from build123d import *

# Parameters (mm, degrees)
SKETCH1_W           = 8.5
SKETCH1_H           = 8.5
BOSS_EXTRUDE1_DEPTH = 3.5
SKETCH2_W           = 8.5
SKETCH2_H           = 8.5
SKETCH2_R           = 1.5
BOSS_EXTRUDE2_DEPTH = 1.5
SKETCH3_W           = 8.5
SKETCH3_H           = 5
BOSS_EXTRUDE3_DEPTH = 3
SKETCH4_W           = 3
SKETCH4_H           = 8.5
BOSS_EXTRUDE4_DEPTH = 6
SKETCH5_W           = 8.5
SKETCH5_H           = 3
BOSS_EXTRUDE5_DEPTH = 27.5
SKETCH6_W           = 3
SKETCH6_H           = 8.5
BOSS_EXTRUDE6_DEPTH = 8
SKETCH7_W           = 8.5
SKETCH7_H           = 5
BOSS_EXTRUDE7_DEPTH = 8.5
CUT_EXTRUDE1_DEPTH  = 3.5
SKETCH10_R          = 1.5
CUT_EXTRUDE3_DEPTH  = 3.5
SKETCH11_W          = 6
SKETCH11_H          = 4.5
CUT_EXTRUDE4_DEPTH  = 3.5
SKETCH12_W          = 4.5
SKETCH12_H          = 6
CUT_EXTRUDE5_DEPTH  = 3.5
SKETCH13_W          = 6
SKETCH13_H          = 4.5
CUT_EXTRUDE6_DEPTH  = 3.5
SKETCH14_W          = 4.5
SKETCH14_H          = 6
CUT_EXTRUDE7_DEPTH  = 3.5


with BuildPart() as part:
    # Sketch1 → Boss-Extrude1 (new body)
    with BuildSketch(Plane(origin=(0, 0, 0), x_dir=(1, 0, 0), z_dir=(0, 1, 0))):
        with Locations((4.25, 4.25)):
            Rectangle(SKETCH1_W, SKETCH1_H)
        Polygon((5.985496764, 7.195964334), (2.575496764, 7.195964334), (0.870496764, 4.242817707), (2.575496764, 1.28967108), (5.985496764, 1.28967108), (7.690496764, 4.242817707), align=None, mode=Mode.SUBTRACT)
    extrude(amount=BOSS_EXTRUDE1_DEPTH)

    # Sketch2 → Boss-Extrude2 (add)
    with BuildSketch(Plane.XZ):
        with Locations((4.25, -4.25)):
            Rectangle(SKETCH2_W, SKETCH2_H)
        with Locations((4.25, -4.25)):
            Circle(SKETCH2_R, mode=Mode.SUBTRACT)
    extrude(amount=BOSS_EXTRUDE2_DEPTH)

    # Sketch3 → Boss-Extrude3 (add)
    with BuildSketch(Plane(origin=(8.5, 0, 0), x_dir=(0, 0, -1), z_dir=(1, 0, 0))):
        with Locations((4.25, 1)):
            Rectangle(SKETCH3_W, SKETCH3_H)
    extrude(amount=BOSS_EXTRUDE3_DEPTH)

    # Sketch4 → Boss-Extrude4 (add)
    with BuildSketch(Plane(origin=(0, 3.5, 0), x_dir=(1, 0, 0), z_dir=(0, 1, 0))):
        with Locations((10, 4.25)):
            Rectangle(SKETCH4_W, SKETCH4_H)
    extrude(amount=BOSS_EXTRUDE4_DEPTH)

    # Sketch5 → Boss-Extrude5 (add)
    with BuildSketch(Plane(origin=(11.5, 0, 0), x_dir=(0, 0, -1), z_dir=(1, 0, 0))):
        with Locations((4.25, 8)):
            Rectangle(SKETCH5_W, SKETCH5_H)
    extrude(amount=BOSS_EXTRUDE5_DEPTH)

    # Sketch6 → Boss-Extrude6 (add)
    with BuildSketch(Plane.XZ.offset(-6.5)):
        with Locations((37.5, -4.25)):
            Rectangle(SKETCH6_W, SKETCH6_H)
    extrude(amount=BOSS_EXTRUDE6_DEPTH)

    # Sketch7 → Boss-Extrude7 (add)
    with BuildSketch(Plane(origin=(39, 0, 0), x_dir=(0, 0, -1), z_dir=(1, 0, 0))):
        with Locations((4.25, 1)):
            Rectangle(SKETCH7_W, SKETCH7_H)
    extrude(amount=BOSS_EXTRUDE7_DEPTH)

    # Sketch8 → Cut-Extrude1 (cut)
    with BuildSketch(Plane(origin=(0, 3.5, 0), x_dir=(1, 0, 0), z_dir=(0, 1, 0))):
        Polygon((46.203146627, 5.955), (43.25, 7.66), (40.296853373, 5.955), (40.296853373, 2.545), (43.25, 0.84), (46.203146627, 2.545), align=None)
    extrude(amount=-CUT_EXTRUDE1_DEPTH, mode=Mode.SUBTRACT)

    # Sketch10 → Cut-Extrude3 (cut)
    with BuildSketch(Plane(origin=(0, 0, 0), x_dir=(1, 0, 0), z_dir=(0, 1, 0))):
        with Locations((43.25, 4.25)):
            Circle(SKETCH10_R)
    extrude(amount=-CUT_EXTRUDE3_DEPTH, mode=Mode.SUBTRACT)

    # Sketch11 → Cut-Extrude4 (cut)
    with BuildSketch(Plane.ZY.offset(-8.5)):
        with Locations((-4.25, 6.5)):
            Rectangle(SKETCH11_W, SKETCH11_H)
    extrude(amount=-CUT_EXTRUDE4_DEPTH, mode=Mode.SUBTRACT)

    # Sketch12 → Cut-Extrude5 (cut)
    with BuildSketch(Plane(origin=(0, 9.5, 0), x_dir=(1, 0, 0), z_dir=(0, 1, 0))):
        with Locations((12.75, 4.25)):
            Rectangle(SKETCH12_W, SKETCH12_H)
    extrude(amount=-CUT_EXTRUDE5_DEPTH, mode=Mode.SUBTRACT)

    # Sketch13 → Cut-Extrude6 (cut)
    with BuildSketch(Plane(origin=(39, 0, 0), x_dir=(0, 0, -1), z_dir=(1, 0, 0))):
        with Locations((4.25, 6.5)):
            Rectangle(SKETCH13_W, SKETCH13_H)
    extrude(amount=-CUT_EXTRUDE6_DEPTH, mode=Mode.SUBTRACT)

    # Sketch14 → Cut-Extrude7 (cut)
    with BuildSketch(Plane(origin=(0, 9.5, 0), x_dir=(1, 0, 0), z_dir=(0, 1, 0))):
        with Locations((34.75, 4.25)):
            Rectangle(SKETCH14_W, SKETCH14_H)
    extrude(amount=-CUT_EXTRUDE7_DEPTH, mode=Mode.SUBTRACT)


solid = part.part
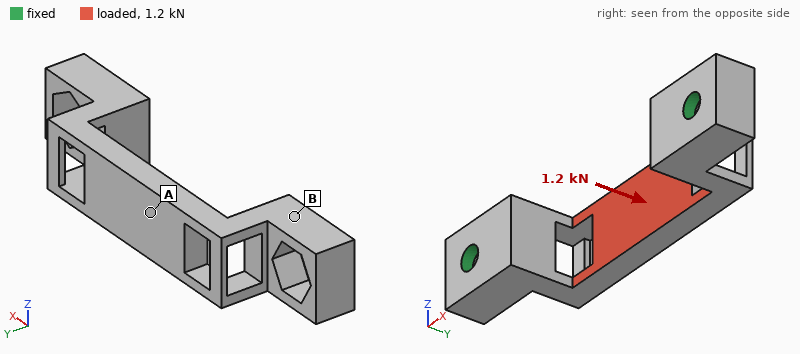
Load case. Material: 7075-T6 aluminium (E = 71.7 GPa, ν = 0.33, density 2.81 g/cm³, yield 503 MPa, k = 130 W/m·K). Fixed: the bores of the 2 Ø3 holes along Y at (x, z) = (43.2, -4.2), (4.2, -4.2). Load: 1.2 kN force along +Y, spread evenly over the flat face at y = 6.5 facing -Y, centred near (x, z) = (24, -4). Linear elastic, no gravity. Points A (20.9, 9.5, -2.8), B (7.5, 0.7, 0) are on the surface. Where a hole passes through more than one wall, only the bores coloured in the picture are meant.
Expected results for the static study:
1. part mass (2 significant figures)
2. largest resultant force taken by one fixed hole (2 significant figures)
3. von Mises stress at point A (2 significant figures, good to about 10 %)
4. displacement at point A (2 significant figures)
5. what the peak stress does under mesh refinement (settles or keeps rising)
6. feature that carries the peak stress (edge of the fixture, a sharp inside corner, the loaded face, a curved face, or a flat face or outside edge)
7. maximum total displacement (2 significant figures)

3.9 g
820 N
220 MPa
0.16 mm
keeps rising
a sharp inside corner
0.17 mm
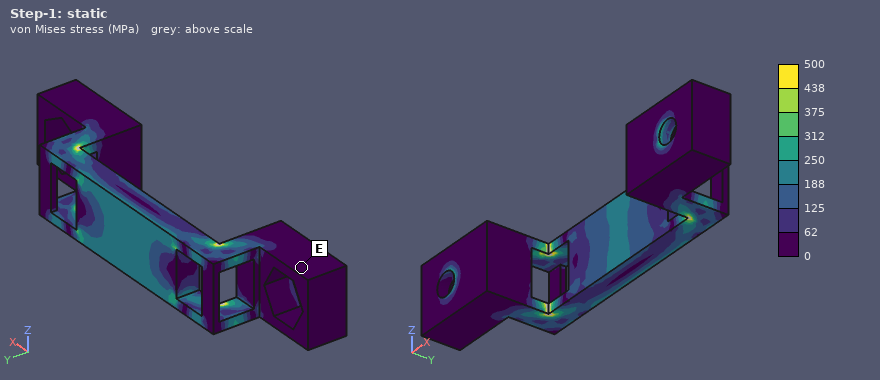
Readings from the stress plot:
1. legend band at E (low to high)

0 to 62 MPa
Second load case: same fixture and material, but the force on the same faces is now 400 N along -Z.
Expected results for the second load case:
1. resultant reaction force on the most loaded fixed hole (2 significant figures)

200 N
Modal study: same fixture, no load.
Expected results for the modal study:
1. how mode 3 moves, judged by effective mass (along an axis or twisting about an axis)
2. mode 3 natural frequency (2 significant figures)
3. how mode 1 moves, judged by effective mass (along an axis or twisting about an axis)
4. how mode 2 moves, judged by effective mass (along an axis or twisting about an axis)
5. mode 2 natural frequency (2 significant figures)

along Y
12 kHz
along Z
along X
11 kHz
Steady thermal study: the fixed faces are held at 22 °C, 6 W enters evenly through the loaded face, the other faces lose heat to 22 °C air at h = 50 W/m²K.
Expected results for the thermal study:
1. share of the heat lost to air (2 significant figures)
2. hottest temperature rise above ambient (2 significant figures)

15 %
33 K
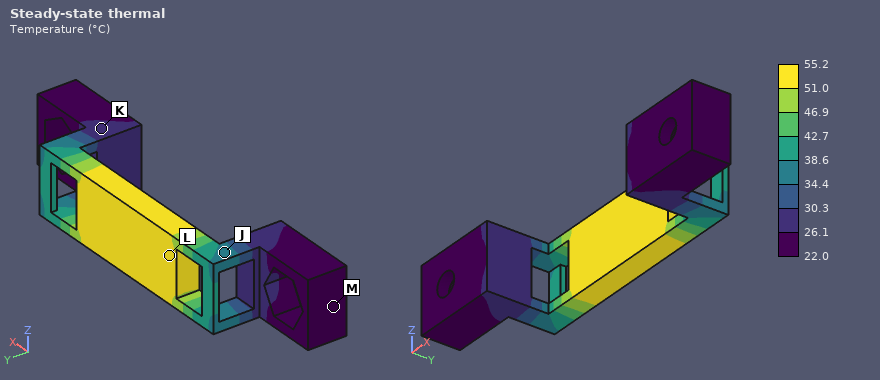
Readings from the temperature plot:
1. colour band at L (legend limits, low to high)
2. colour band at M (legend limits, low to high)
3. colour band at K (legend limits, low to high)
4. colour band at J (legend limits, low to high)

51.0 to 55.2 °C
22.0 to 26.1 °C
26.1 to 30.3 °C
34.4 to 38.6 °C
